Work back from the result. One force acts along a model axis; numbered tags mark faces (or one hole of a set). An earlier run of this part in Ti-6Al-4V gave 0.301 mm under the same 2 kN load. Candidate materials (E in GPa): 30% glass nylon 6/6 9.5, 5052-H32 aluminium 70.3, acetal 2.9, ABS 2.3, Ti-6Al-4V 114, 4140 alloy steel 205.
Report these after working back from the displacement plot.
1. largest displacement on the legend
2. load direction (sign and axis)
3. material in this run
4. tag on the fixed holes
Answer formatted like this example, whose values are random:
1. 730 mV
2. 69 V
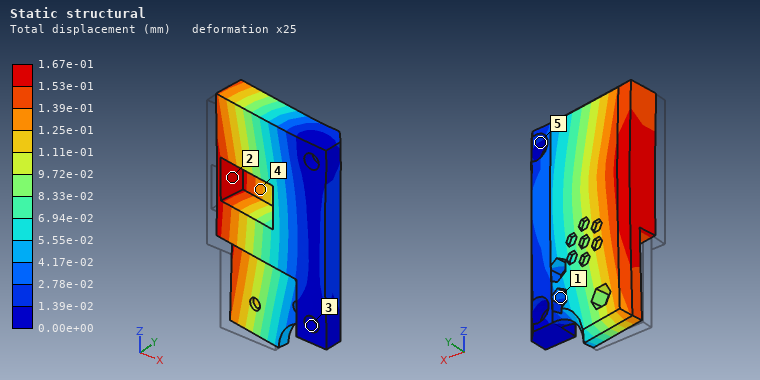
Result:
1. 1.67e-01 mm
2. +Y
3. 4140 alloy steel
4. 3
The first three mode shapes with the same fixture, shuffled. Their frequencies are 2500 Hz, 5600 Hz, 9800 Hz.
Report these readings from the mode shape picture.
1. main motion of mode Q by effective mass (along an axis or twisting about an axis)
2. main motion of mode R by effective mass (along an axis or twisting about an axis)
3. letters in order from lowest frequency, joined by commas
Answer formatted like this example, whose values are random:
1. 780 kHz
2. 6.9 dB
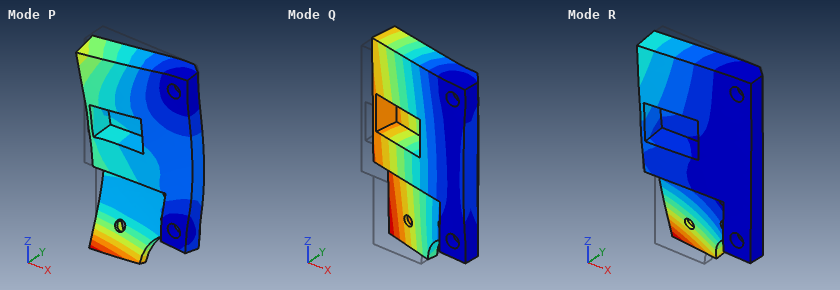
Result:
1. along Y
2. twisting about X
3. Q, R, P
